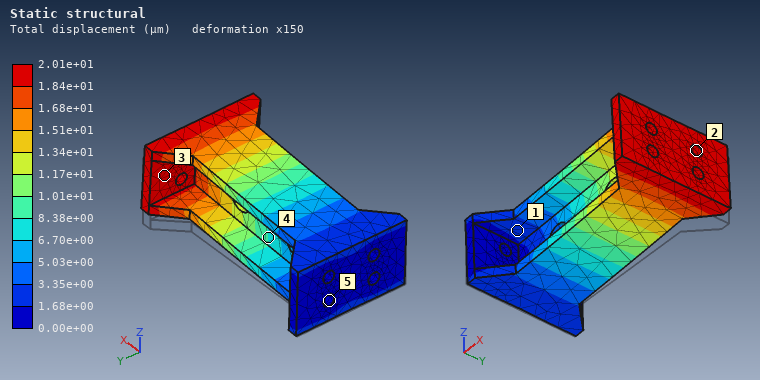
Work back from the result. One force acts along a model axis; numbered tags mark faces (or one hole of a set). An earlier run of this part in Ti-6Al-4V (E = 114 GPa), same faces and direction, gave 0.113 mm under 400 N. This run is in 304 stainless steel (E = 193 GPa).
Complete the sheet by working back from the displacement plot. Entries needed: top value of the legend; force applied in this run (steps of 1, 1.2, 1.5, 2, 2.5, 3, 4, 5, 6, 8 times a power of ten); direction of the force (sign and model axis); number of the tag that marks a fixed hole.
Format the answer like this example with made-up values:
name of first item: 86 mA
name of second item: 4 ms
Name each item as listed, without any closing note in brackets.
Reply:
top value of the legend: 2.01e+01 µm
force applied in this run: 120 N
direction of the force: +Z
number of the tag that marks a fixed hole: 5
